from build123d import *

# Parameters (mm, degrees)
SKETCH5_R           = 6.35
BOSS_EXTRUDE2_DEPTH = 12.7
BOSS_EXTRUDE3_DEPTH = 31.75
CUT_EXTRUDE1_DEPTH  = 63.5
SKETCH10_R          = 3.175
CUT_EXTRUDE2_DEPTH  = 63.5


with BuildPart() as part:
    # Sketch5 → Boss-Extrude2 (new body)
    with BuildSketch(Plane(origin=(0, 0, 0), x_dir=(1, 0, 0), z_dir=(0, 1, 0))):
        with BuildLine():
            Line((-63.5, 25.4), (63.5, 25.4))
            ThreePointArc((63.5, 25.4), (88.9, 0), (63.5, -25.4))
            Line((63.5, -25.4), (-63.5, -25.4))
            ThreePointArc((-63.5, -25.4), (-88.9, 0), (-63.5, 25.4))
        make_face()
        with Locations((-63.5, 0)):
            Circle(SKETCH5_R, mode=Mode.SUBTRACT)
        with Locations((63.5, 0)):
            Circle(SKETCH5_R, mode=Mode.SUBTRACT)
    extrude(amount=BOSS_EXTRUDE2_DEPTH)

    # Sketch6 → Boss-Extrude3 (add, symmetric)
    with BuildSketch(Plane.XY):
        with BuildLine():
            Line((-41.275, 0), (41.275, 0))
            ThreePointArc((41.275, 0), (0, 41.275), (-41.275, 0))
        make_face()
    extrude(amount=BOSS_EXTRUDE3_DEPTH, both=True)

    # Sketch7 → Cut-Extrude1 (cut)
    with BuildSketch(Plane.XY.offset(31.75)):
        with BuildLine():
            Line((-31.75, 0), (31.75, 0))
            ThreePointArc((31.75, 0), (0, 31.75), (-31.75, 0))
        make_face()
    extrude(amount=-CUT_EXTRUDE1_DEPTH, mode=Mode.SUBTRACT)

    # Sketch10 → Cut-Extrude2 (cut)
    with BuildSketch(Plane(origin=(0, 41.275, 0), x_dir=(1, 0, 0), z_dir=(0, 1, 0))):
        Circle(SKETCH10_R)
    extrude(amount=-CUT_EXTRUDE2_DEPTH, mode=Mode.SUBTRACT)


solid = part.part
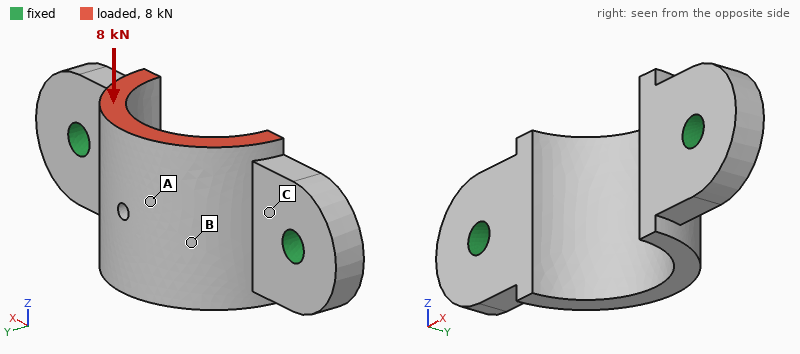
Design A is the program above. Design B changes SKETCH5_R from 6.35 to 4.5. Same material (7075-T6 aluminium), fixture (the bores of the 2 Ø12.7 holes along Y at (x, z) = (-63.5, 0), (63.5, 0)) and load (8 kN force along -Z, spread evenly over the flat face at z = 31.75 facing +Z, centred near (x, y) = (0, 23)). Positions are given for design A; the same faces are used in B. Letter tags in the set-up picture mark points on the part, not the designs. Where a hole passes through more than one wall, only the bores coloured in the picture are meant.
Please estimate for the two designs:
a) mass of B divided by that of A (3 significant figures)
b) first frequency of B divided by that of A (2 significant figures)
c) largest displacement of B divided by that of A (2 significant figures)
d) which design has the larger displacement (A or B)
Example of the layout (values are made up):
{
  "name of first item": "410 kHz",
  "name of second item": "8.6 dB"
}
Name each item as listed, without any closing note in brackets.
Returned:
{
  "mass of B divided by that of A": "1.01",
  "first frequency of B divided by that of A": "0.86",
  "largest displacement of B divided by that of A": "1.4",
  "which design has the larger displacement": "B"
}
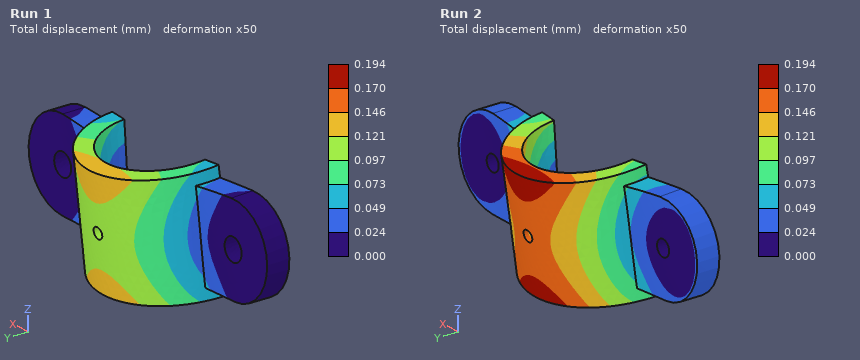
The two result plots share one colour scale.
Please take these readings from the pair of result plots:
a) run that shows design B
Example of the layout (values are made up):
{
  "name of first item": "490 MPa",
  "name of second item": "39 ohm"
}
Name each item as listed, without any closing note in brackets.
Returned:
{
  "run that shows design B": "Run 2"
}
